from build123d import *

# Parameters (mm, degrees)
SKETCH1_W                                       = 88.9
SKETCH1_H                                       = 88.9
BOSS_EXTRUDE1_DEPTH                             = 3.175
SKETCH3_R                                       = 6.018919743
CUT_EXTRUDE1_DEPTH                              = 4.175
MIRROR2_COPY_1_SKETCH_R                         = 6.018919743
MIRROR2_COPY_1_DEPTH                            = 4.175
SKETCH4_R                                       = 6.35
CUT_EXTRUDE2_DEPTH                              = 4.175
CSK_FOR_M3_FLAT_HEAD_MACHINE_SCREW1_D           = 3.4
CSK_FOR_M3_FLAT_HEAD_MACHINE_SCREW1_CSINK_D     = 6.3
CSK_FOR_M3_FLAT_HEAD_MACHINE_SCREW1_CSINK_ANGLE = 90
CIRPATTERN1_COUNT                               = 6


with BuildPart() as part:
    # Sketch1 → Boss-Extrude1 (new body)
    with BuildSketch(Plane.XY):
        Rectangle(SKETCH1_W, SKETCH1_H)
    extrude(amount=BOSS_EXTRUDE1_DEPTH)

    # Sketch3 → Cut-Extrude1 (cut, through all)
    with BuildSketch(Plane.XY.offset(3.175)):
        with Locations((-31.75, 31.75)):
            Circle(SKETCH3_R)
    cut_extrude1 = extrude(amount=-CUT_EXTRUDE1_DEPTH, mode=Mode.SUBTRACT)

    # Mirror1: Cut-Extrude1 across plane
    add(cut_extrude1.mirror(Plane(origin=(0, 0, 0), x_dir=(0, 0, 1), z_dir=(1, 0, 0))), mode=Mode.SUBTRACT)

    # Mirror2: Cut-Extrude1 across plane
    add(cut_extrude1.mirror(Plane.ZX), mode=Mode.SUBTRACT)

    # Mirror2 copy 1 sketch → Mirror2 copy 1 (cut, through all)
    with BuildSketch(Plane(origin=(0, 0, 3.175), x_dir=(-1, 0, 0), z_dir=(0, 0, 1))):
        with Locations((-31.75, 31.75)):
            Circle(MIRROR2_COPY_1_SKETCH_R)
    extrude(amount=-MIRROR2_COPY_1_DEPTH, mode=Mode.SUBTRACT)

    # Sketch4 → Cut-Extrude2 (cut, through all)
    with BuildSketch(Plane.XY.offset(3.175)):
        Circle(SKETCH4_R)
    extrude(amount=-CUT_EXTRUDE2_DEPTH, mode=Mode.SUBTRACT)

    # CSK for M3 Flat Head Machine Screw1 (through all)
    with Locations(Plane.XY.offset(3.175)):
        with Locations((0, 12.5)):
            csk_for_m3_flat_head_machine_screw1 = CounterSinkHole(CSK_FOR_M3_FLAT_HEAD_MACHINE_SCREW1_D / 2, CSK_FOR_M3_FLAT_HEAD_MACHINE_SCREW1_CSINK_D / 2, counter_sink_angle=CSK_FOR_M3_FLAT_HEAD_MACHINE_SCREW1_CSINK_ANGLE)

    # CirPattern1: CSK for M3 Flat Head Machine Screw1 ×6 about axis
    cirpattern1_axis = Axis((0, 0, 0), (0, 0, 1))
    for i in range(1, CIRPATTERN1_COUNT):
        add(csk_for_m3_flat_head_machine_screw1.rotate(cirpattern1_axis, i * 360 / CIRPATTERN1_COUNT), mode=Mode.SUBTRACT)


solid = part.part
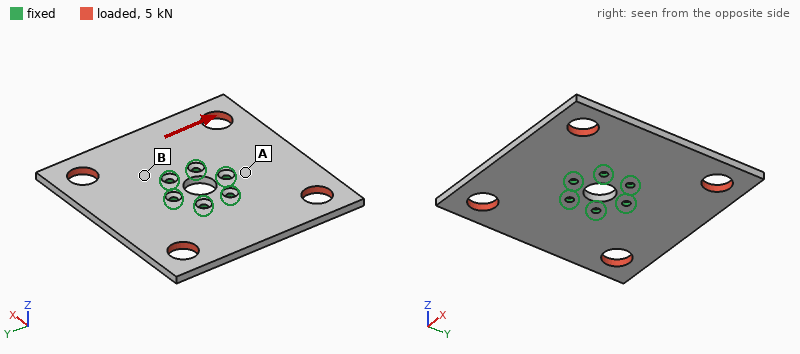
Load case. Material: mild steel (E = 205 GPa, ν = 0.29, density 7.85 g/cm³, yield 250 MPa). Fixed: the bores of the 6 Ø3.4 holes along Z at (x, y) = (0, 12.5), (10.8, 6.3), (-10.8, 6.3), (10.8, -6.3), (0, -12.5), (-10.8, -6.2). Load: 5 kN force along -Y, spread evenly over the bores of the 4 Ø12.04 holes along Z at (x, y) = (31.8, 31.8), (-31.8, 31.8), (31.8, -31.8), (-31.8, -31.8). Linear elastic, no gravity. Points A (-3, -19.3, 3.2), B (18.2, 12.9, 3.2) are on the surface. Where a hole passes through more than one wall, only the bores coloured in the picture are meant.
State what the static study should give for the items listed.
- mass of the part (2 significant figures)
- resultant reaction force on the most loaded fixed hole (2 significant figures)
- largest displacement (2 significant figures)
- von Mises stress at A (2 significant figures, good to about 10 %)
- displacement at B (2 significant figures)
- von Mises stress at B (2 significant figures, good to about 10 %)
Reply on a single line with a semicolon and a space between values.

180 g; 970 N; 8.4 µm; 12 MPa; 2.3 µm; 19 MPa
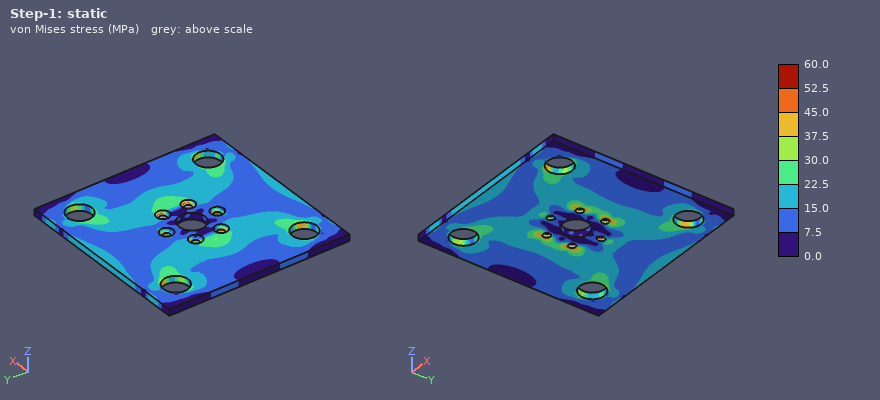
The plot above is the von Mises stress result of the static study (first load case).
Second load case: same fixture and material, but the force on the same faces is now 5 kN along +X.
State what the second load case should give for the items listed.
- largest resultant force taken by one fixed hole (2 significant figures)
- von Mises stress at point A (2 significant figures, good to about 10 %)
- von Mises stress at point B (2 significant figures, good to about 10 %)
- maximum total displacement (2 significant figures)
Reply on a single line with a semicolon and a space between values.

1.1 kN; 22 MPa; 17 MPa; 8.4 µm
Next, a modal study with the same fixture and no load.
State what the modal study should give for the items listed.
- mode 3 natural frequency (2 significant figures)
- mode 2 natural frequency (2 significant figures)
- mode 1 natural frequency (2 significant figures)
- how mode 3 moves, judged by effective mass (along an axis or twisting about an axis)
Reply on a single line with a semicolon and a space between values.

1600 Hz; 1500 Hz; 1500 Hz; along Z
